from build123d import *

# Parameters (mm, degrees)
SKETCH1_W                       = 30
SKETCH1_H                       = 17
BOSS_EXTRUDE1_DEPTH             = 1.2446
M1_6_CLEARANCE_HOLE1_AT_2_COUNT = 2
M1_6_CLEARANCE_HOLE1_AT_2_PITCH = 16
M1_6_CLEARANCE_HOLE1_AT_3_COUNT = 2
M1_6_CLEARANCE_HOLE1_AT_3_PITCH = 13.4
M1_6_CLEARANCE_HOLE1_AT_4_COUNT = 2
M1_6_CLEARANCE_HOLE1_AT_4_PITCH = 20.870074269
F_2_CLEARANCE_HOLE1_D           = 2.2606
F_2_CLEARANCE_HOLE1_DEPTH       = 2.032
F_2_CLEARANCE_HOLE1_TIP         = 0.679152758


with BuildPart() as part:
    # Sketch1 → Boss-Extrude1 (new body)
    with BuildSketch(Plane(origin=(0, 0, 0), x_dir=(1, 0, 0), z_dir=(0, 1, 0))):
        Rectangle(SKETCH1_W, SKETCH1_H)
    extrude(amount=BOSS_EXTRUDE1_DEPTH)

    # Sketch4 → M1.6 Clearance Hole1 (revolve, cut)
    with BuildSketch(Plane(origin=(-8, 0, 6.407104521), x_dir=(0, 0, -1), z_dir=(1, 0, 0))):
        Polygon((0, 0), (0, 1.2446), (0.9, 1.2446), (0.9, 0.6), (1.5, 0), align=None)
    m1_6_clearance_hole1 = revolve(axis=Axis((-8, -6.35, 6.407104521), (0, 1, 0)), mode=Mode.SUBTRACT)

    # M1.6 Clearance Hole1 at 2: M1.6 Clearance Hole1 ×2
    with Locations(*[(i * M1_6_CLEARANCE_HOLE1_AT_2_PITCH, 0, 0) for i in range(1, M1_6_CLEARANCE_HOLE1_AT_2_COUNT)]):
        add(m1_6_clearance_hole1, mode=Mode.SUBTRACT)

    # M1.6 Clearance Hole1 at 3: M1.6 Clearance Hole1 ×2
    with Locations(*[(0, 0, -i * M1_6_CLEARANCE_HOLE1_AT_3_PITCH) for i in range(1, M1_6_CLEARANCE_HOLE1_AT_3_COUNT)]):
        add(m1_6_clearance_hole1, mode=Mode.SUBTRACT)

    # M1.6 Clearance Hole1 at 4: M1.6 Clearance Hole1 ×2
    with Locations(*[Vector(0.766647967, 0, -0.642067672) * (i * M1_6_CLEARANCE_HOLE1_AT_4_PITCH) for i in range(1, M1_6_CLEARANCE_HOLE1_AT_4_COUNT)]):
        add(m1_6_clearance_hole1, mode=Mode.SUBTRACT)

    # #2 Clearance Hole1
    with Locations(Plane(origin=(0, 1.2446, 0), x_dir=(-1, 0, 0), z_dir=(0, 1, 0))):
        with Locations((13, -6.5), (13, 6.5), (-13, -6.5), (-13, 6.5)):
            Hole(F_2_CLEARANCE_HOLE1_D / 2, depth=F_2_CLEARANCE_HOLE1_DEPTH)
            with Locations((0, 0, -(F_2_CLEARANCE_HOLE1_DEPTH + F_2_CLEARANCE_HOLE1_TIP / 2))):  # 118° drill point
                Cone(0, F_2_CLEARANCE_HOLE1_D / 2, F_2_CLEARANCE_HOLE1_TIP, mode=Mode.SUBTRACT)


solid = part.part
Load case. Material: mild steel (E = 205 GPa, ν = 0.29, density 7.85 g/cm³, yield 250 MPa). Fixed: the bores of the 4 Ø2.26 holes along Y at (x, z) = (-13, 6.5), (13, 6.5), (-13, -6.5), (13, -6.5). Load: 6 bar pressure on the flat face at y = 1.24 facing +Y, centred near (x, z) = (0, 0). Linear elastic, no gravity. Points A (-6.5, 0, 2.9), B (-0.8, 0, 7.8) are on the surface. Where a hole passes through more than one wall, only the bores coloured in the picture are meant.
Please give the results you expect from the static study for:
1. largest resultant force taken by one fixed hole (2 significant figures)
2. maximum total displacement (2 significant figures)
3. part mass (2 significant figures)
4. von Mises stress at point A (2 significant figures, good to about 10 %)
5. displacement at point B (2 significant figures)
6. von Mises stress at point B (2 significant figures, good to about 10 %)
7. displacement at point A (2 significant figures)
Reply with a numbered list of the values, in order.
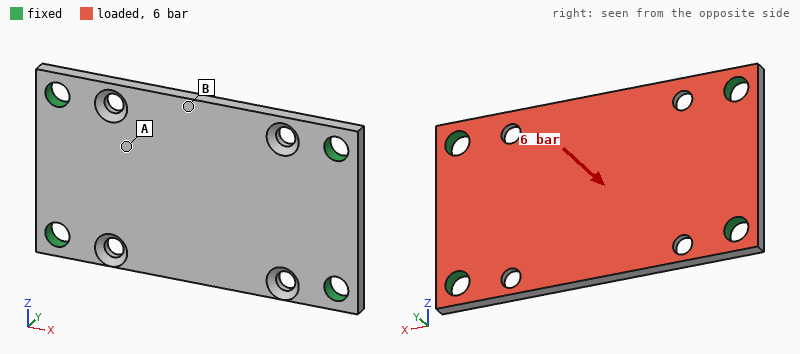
1. 73 N
2. 22 µm
3. 4.7 g
4. 21 MPa
5. 21 µm
6. 69 MPa
7. 13 µm
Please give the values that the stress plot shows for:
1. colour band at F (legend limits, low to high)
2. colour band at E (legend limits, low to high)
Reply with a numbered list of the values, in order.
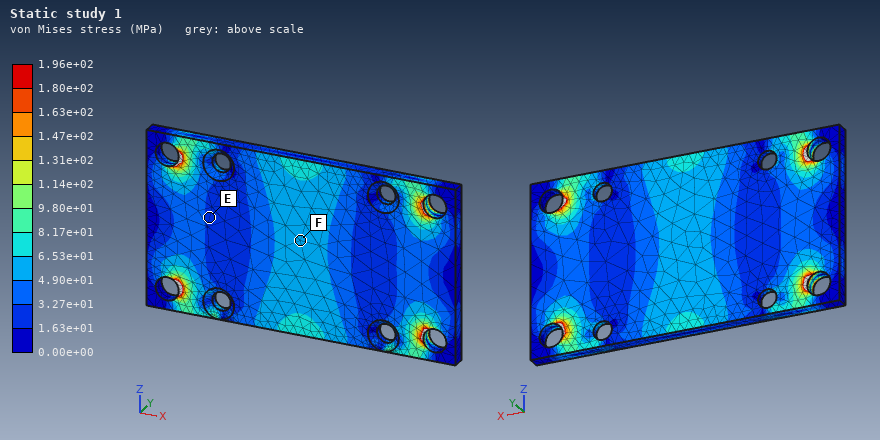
1. 4.90e+01 to 6.53e+01 MPa
2. 1.63e+01 to 3.27e+01 MPa
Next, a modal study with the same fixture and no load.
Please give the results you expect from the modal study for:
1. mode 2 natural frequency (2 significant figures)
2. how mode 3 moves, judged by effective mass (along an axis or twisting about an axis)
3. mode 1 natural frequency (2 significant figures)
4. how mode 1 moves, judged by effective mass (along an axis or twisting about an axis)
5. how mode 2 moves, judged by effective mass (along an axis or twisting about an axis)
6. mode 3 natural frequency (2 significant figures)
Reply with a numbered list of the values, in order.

1. 14 kHz
2. twisting about Z
3. 9700 Hz
4. along Y
5. twisting about X
6. 26 kHz
